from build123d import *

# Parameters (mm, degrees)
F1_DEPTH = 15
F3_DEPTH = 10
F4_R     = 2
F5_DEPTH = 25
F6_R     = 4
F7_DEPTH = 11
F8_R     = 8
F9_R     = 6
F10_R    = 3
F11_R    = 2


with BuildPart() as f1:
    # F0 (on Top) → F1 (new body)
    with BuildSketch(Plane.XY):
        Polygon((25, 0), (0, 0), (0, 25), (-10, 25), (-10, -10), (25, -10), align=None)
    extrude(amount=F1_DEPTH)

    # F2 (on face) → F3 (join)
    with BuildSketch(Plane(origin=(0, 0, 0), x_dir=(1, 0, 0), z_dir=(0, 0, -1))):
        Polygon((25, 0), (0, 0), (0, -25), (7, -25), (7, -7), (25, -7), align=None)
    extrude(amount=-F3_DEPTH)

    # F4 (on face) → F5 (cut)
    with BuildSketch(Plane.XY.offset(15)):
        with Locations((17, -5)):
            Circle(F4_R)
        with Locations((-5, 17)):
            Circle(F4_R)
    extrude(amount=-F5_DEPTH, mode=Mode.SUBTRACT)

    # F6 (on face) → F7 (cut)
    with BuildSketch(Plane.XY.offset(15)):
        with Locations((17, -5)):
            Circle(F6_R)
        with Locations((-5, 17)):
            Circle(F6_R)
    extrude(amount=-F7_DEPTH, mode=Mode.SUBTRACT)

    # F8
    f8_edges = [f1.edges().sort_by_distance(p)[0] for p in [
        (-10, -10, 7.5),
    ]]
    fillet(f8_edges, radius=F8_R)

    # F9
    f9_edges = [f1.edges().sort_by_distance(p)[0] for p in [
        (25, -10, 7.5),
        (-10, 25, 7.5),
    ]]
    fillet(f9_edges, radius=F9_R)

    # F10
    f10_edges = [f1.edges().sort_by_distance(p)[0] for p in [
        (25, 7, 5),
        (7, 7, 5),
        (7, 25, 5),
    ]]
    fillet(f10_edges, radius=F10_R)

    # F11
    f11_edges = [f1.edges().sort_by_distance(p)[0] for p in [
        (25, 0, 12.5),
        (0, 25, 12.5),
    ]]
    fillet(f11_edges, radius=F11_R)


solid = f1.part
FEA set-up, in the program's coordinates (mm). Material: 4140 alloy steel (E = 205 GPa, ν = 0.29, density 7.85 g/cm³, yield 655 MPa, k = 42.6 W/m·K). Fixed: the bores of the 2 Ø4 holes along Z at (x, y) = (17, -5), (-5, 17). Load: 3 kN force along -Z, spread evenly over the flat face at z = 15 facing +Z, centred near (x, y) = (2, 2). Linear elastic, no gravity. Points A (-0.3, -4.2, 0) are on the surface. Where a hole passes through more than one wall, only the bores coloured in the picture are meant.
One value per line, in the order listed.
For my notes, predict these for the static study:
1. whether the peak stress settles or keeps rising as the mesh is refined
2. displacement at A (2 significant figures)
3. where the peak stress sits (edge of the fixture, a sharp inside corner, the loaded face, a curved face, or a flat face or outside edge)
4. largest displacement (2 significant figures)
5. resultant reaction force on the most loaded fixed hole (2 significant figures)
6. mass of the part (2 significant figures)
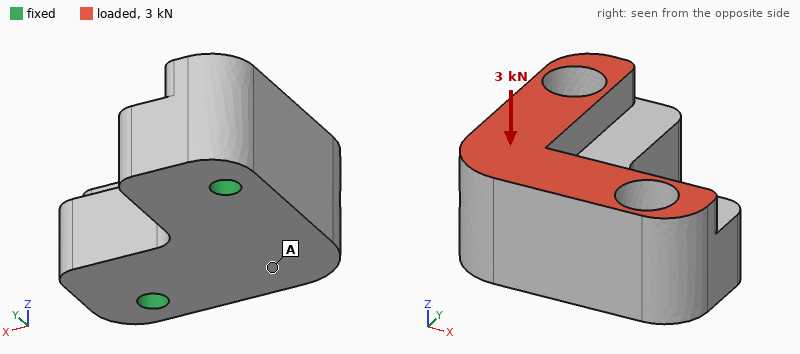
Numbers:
keeps rising
14 µm
edge of the fixture
25 µm
1.6 kN
81 g
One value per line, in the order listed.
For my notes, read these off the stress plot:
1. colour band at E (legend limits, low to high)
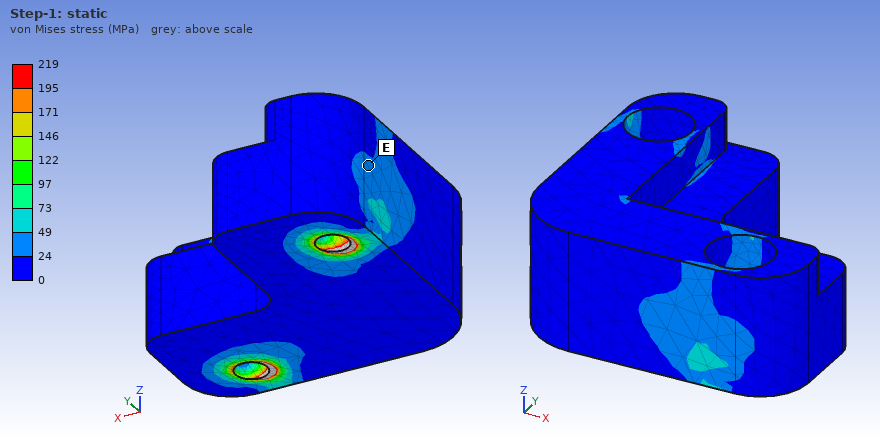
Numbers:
24 to 49 MPa
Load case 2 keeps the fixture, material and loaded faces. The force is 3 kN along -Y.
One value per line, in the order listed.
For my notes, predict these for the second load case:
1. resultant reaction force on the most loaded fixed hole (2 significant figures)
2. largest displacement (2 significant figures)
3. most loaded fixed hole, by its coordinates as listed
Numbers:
2.1 kN
33 µm
(-5, 17)
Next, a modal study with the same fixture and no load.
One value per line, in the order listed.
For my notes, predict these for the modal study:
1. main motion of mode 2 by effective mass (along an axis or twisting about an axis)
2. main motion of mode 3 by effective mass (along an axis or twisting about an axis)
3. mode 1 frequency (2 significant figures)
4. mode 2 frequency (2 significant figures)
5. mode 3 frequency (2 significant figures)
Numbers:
along Z
twisting about Z
7700 Hz
21 kHz
24 kHz
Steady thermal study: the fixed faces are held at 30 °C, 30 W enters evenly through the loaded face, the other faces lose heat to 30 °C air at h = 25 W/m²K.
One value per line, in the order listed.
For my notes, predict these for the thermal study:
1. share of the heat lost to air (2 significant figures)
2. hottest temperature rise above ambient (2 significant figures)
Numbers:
7.1 %
44 K
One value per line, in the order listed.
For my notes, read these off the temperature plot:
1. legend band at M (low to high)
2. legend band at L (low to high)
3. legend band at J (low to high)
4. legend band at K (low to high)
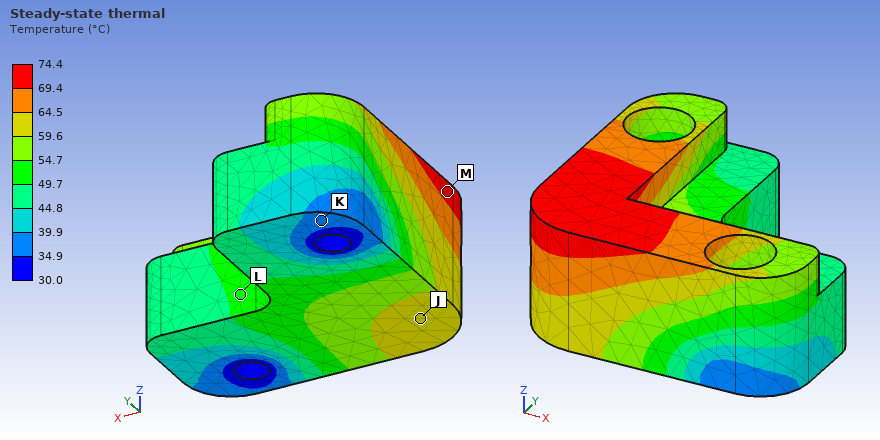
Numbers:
69.4 to 74.4 °C
49.7 to 54.7 °C
59.6 to 64.5 °C
34.9 to 39.9 °C
